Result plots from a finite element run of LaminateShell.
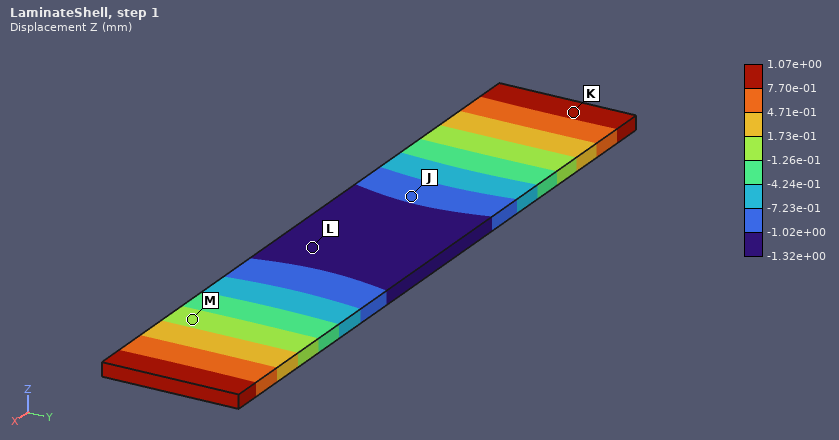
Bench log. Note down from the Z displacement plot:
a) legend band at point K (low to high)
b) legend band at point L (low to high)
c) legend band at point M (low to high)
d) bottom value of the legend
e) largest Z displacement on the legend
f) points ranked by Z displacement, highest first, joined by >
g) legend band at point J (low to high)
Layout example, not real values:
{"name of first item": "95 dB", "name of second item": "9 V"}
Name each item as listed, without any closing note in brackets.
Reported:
{"legend band at point K": "7.70e-01 to 1.07e+00 mm", "legend band at point L": "-1.32e+00 to -1.02e+00 mm", "legend band at point M": "-1.26e-01 to 1.73e-01 mm", "bottom value of the legend": "-1.32e+00 mm", "largest Z displacement on the legend": "1.07e+00 mm", "points ranked by Z displacement, highest first, joined by >": "K > M > J > L", "legend band at point J": "-1.02e+00 to -7.23e-01 mm"}
